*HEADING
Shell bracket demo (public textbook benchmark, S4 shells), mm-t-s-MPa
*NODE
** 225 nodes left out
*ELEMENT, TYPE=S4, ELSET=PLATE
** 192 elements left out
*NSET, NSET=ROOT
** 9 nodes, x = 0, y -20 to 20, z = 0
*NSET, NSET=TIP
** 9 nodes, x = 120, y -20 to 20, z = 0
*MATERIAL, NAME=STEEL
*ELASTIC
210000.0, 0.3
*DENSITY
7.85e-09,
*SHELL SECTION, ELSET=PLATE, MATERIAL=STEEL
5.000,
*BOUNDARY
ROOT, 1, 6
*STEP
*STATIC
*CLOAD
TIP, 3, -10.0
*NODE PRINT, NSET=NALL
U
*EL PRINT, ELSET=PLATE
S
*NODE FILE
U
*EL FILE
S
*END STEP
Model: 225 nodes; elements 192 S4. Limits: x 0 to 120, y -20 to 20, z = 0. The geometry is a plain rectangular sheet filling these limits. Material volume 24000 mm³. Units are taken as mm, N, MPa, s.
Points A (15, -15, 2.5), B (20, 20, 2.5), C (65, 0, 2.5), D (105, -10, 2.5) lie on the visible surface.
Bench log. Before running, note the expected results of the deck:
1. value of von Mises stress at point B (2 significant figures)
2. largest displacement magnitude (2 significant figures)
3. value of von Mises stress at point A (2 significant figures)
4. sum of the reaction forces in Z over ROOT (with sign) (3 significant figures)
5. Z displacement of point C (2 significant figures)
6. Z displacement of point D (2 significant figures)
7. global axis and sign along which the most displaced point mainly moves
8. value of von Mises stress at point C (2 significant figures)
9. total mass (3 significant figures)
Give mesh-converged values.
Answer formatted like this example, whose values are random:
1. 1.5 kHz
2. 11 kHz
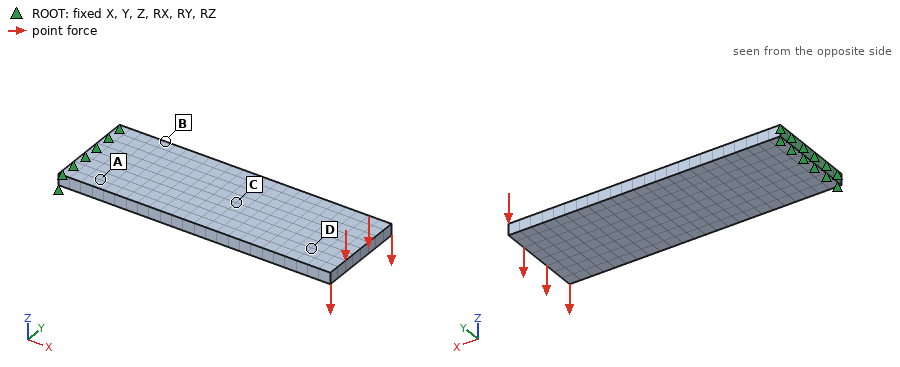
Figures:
1. 55 MPa
2. 0.57 mm
3. 57 MPa
4. 90.0 N
5. -0.21 mm
6. -0.47 mm
7. -Z
8. 30 MPa
9. 0.188 kg
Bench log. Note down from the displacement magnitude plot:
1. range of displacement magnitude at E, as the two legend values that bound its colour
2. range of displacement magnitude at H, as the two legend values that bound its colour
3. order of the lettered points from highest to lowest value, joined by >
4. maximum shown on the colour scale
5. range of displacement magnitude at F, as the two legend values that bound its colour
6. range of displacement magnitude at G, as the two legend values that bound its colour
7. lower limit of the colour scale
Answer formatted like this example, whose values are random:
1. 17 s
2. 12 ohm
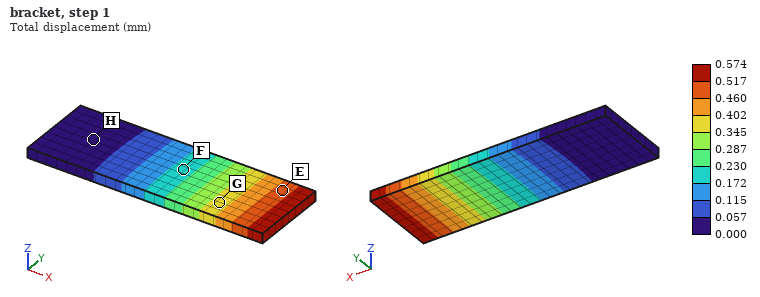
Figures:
1. 0.460 to 0.517 mm
2. 0.000 to 0.057 mm
3. E > G > F > H
4. 0.574 mm
5. 0.172 to 0.230 mm
6. 0.345 to 0.402 mm
7. 0.000 mm
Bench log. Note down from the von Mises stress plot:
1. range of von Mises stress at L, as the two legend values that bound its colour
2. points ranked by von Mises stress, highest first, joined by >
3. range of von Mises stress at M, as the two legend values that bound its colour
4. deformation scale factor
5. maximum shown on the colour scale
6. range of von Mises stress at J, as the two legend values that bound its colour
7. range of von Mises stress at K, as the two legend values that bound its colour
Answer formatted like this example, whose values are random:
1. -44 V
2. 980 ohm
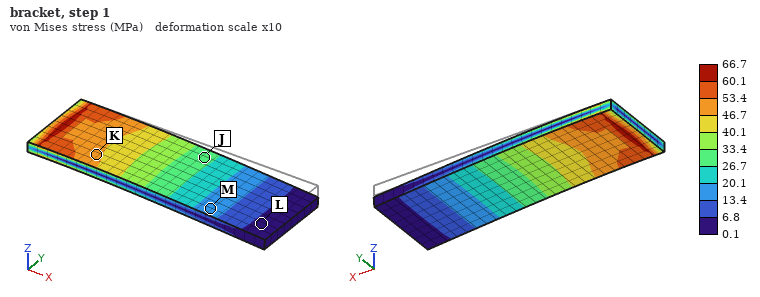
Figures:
1. 0.1 to 6.8 MPa
2. K > J > M > L
3. 13.4 to 20.1 MPa
4. 10
5. 66.7 MPa
6. 26.7 to 33.4 MPa
7. 46.7 to 53.4 MPa
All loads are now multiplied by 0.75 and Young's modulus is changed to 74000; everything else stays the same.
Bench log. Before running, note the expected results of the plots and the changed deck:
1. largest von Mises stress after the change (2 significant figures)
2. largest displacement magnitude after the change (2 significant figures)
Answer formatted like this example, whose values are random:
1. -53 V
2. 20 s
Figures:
1. 50 MPa
2. 1.2 mm
